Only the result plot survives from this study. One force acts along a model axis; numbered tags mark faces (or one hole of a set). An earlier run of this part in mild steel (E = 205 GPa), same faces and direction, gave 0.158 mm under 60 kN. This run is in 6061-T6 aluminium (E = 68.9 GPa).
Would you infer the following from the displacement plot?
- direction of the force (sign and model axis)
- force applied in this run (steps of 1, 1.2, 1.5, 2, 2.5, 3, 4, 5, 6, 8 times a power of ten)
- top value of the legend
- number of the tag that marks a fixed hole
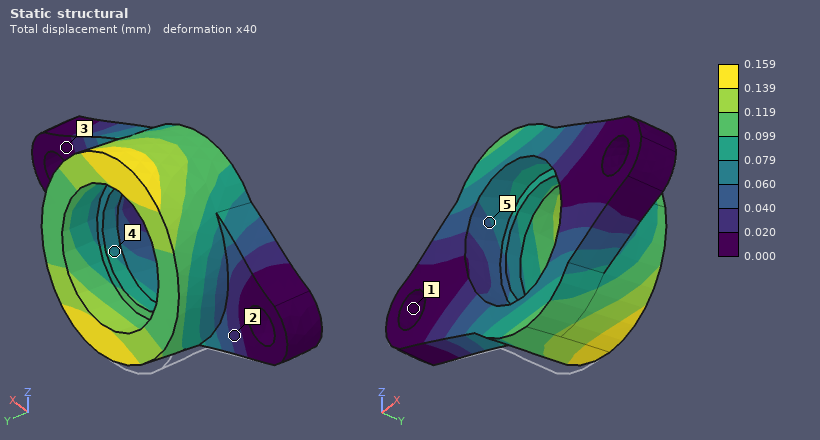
+Z
20 kN
0.159 mm
1
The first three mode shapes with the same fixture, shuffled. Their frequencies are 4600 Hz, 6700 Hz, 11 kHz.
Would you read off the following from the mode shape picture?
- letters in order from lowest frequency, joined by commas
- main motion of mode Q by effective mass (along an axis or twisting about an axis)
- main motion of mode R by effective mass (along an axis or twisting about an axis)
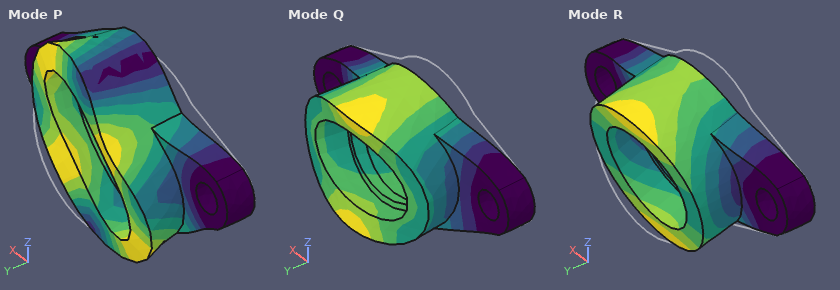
R, Q, P
along Y
along Z
